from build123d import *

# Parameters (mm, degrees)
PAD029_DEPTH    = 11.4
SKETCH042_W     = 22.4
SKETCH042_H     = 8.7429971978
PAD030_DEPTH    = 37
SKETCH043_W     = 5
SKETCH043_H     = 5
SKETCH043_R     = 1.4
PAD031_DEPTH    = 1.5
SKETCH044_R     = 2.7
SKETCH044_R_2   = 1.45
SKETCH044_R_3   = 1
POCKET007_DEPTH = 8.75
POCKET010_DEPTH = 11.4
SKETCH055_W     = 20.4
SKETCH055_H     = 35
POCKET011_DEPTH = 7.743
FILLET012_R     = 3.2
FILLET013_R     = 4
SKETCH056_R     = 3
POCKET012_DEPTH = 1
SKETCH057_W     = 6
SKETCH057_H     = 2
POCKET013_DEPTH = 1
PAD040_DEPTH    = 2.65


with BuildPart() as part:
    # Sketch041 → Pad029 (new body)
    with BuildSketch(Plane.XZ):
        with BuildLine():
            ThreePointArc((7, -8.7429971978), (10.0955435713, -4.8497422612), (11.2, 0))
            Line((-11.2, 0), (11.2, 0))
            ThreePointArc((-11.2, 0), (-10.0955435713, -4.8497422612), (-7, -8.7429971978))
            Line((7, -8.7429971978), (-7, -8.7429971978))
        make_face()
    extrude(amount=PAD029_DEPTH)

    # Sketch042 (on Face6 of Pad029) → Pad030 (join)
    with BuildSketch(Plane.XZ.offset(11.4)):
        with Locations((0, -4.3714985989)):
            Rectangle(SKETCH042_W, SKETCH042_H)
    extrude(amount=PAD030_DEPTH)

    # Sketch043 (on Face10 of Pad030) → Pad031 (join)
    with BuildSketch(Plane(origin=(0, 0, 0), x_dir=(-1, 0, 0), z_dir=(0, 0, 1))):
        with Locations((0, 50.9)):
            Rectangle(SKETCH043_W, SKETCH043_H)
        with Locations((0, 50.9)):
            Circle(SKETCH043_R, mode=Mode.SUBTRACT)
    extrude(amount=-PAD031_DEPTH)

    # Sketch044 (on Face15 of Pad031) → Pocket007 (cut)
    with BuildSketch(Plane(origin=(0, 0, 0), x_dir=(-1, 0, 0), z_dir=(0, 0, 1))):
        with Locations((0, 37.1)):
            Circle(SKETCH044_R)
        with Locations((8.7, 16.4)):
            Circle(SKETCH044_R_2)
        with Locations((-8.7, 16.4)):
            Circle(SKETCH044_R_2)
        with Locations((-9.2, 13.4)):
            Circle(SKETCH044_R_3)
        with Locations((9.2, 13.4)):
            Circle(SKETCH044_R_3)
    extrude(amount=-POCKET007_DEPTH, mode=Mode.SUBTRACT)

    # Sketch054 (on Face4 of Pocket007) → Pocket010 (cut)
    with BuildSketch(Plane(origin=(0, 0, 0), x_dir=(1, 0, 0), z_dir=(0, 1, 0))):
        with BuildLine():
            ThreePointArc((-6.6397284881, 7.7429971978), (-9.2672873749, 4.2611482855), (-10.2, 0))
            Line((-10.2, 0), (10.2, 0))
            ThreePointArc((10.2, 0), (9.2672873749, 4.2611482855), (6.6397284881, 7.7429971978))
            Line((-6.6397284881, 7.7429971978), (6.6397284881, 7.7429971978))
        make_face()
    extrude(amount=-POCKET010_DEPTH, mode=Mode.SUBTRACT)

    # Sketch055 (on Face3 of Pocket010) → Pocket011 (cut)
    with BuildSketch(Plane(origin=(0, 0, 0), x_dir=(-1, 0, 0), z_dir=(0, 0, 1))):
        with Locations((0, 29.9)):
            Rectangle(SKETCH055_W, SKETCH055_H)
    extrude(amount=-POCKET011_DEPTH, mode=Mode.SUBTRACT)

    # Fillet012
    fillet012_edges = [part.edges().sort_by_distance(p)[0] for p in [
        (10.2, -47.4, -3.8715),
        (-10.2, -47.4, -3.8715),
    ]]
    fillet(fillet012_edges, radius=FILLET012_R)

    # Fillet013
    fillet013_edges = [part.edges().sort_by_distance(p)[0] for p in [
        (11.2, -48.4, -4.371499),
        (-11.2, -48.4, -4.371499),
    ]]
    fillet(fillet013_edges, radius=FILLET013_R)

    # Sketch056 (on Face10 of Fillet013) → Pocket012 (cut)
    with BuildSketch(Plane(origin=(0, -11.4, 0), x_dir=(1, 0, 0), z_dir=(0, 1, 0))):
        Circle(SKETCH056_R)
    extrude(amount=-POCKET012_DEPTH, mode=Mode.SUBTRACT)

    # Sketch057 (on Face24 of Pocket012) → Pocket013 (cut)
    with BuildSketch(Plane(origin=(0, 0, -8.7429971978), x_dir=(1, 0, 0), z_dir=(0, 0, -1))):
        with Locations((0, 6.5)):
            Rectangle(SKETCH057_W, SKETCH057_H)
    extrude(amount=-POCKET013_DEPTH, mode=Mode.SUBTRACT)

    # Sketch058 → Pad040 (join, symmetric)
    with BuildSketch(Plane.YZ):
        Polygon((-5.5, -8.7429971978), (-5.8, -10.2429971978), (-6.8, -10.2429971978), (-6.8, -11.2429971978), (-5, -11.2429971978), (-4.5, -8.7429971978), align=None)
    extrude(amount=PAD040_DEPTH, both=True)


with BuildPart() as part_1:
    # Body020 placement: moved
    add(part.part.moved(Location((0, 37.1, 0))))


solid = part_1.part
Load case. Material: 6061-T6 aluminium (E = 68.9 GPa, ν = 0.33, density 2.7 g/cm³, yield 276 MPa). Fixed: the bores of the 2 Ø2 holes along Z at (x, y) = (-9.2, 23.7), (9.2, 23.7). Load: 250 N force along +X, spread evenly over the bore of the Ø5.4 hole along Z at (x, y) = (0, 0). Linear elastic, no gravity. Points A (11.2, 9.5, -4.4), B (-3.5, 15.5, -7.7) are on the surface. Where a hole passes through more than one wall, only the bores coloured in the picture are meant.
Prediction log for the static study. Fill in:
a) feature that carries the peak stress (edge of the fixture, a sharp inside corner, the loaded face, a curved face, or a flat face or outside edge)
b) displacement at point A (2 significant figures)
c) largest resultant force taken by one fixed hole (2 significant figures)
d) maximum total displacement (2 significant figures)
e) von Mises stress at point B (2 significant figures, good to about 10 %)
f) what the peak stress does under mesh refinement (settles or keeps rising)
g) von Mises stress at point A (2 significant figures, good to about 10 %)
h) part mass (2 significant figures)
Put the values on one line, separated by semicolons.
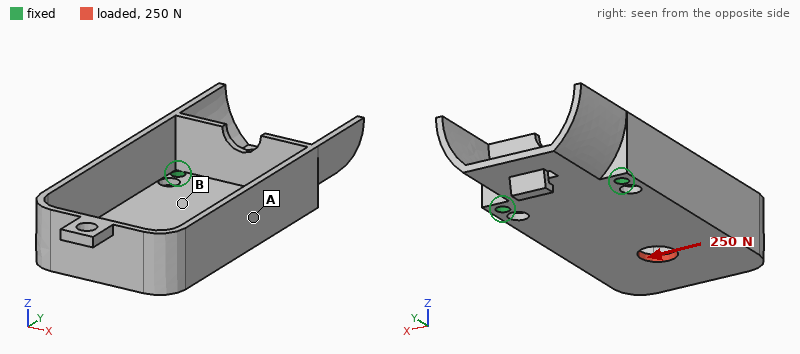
edge of the fixture; 22 µm; 330 N; 71 µm; 27 MPa; keeps rising; 10 MPa; 5.5 g
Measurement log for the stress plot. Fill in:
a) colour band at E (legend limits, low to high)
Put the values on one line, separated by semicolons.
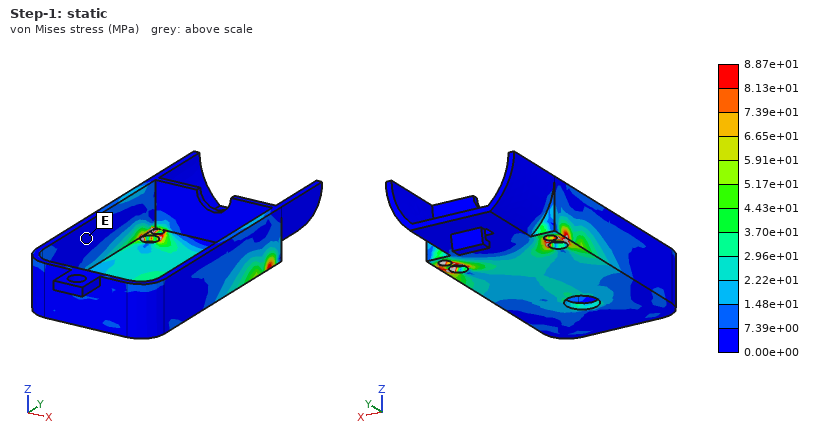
0.00e+00 to 7.39e+00 MPa
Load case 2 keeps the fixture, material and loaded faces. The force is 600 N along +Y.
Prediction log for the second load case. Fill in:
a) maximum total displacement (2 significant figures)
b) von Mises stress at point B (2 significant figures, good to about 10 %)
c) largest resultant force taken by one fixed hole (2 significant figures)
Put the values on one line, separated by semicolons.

56 µm; 21 MPa; 300 N
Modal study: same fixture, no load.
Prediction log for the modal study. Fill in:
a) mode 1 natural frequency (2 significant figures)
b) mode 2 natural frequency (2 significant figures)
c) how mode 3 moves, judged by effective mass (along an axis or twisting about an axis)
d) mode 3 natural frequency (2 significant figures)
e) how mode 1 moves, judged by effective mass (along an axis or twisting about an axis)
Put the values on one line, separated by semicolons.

1500 Hz; 2600 Hz; along X; 7500 Hz; along Z
